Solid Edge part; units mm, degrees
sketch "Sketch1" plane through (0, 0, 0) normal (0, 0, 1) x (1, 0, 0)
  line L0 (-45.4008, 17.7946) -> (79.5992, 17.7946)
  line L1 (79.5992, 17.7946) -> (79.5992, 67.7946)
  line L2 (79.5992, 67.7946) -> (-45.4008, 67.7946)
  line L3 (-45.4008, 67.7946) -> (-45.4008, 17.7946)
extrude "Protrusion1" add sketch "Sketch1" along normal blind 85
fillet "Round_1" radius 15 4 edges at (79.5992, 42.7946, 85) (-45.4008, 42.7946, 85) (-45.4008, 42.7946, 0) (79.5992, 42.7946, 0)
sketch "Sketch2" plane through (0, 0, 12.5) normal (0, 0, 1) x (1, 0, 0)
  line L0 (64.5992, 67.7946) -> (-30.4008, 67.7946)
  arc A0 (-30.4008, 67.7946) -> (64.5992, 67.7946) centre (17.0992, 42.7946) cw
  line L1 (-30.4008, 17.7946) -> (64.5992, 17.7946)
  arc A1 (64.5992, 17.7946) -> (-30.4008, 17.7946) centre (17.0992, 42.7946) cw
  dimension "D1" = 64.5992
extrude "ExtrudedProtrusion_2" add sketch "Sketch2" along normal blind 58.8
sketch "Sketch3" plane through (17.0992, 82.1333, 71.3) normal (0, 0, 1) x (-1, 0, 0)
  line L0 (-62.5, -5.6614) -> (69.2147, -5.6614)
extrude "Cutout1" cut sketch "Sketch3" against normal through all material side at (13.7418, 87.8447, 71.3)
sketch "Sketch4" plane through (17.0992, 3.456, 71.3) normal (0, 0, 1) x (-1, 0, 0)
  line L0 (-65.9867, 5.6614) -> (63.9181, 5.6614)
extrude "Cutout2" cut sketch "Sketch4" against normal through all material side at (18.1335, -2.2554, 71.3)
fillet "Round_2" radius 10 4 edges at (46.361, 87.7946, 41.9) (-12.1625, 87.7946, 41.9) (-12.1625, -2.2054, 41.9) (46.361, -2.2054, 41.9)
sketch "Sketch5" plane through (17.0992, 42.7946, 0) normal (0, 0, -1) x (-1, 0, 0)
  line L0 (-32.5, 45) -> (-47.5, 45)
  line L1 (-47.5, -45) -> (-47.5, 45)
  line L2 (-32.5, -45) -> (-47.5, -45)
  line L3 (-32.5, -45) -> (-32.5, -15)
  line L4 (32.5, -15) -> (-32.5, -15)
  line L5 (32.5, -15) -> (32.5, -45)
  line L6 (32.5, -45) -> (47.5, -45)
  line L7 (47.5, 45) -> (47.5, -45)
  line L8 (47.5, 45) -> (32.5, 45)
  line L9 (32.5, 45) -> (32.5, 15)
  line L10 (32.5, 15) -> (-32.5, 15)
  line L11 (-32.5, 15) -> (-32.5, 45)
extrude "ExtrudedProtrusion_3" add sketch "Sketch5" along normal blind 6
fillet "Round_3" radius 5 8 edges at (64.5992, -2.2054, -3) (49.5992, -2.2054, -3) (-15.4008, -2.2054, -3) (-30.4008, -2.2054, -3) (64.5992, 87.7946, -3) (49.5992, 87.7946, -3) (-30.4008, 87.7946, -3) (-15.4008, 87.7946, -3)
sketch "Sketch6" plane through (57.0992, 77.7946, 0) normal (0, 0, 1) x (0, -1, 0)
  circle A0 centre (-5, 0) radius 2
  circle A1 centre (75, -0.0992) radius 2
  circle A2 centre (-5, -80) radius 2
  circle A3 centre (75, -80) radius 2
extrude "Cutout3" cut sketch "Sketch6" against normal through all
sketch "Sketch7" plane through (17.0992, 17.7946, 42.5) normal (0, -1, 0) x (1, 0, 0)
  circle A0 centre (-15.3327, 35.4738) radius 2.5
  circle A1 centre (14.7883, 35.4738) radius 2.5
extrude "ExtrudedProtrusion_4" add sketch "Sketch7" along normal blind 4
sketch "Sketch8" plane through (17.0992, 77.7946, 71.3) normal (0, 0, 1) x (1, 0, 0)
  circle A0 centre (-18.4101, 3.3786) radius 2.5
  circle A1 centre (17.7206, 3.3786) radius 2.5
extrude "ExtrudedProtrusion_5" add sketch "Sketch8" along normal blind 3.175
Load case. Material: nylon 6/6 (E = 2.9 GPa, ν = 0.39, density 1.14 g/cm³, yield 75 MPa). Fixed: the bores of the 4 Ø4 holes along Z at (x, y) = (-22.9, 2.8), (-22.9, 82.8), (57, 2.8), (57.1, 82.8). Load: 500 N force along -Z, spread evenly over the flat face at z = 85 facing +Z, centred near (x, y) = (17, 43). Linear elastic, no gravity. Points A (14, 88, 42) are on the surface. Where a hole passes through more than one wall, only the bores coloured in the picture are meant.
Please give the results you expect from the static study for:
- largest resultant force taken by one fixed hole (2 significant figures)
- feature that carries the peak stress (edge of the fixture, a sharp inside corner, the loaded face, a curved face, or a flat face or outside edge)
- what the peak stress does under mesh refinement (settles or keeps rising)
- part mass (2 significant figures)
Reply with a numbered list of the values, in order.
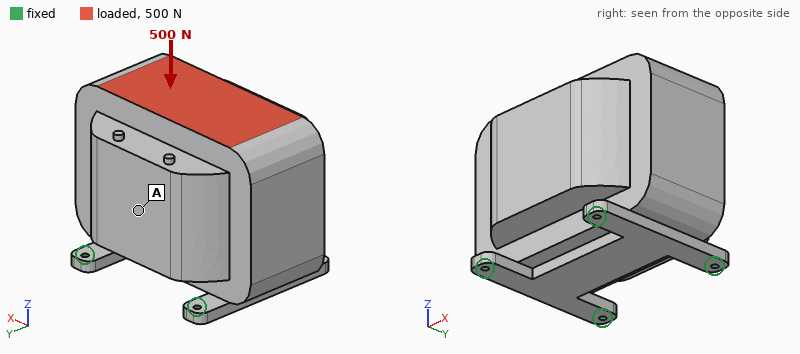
1. 140 N
2. edge of the fixture
3. keeps rising
4. 840 g
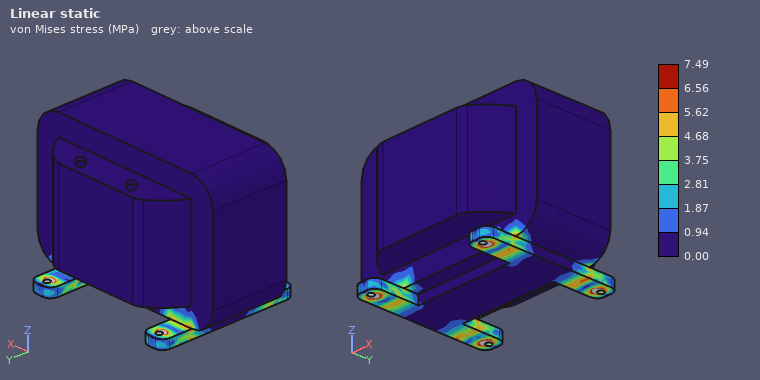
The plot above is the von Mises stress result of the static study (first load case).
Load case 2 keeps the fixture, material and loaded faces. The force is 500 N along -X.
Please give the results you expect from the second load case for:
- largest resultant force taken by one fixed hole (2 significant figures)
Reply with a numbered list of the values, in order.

1. 330 N
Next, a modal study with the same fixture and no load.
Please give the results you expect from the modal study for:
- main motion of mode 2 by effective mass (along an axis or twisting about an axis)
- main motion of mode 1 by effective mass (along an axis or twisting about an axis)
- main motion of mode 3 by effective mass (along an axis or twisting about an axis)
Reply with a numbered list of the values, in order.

1. along X
2. along Y
3. along Z
